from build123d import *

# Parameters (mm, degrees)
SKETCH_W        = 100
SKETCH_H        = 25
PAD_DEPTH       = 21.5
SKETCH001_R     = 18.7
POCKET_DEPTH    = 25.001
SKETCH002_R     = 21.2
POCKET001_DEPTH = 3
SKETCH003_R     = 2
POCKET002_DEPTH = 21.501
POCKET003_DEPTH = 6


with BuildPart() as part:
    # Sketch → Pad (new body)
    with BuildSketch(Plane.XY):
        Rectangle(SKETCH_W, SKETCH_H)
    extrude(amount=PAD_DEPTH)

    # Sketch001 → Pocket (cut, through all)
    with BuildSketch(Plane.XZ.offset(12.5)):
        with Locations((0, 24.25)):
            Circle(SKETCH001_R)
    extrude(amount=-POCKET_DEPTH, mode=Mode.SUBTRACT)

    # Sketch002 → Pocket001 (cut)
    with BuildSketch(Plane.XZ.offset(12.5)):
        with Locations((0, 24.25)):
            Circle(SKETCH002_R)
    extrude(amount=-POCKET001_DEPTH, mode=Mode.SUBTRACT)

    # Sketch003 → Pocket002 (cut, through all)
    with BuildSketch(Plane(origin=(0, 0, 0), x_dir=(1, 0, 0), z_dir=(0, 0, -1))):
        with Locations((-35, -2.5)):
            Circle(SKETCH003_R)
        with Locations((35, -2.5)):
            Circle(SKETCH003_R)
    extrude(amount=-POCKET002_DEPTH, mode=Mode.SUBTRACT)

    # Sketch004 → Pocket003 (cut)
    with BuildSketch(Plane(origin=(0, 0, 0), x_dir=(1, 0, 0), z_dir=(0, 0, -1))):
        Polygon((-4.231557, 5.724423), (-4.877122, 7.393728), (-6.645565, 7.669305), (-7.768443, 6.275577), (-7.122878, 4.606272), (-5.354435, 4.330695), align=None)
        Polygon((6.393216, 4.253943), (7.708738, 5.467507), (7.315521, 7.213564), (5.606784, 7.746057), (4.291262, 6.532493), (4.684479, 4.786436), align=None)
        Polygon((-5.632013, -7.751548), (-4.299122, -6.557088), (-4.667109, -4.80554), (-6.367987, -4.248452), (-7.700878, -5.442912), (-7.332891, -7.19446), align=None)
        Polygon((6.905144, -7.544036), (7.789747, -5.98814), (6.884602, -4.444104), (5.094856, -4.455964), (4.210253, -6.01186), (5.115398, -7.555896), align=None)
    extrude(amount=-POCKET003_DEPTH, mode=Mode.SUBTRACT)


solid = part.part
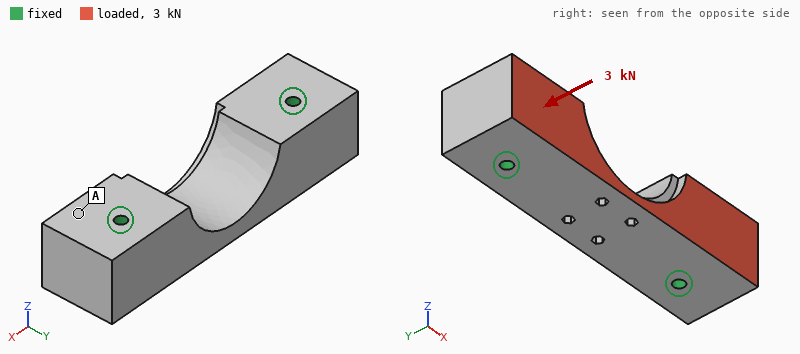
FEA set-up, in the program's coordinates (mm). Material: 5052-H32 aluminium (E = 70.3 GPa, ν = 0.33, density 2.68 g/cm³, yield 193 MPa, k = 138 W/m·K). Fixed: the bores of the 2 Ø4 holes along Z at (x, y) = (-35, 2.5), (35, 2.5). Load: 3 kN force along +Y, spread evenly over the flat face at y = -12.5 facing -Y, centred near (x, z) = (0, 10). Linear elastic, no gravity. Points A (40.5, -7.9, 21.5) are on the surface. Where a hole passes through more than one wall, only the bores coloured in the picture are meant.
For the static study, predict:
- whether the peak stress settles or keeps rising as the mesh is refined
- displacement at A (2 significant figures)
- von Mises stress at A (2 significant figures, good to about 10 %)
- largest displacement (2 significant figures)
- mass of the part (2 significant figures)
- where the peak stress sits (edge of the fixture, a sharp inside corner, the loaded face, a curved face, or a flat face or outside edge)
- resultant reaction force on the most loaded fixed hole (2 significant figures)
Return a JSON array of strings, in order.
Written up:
["keeps rising", "0.78 µm", "2.7 MPa", "5.2 µm", "110 g", "edge of the fixture", "1.5 kN"]
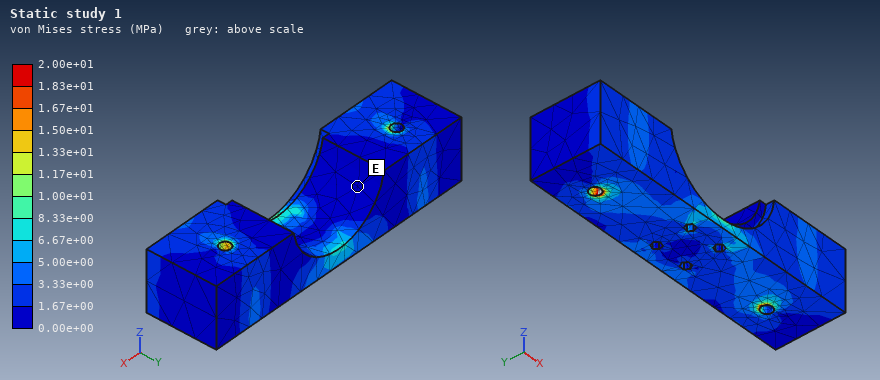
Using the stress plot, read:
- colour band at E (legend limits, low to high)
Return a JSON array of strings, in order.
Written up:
["0.00e+00 to 1.67e+00 MPa"]
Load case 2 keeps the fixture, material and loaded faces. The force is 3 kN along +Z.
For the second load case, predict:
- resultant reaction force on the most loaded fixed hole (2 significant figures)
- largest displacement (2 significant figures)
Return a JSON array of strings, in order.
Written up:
["1.5 kN", "9.6 µm"]
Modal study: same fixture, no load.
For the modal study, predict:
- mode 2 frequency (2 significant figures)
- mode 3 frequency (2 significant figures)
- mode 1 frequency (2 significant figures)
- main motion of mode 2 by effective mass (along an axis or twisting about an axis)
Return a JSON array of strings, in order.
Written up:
["17 kHz", "19 kHz", "10 kHz", "along Z"]
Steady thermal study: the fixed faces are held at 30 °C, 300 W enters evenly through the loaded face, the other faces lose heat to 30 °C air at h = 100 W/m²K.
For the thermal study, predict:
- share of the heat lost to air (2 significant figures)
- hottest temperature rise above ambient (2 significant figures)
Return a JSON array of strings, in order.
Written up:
["4.6 %", "35 K"]
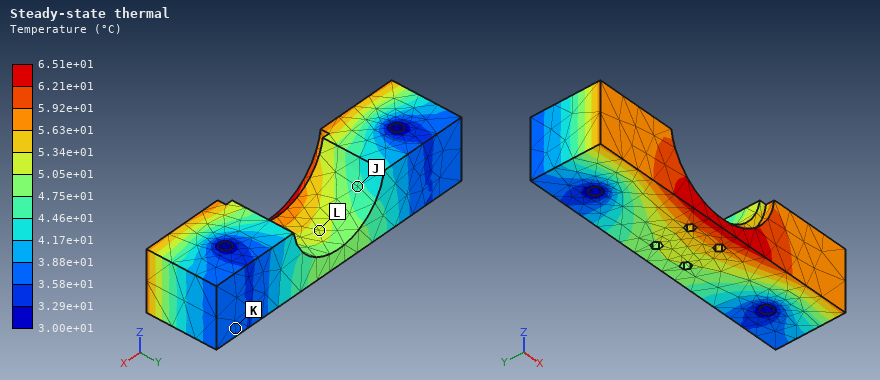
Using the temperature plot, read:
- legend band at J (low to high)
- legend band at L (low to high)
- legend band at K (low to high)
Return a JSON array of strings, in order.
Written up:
["4.46e+01 to 4.75e+01 °C", "5.05e+01 to 5.34e+01 °C", "3.58e+01 to 3.88e+01 °C"]
